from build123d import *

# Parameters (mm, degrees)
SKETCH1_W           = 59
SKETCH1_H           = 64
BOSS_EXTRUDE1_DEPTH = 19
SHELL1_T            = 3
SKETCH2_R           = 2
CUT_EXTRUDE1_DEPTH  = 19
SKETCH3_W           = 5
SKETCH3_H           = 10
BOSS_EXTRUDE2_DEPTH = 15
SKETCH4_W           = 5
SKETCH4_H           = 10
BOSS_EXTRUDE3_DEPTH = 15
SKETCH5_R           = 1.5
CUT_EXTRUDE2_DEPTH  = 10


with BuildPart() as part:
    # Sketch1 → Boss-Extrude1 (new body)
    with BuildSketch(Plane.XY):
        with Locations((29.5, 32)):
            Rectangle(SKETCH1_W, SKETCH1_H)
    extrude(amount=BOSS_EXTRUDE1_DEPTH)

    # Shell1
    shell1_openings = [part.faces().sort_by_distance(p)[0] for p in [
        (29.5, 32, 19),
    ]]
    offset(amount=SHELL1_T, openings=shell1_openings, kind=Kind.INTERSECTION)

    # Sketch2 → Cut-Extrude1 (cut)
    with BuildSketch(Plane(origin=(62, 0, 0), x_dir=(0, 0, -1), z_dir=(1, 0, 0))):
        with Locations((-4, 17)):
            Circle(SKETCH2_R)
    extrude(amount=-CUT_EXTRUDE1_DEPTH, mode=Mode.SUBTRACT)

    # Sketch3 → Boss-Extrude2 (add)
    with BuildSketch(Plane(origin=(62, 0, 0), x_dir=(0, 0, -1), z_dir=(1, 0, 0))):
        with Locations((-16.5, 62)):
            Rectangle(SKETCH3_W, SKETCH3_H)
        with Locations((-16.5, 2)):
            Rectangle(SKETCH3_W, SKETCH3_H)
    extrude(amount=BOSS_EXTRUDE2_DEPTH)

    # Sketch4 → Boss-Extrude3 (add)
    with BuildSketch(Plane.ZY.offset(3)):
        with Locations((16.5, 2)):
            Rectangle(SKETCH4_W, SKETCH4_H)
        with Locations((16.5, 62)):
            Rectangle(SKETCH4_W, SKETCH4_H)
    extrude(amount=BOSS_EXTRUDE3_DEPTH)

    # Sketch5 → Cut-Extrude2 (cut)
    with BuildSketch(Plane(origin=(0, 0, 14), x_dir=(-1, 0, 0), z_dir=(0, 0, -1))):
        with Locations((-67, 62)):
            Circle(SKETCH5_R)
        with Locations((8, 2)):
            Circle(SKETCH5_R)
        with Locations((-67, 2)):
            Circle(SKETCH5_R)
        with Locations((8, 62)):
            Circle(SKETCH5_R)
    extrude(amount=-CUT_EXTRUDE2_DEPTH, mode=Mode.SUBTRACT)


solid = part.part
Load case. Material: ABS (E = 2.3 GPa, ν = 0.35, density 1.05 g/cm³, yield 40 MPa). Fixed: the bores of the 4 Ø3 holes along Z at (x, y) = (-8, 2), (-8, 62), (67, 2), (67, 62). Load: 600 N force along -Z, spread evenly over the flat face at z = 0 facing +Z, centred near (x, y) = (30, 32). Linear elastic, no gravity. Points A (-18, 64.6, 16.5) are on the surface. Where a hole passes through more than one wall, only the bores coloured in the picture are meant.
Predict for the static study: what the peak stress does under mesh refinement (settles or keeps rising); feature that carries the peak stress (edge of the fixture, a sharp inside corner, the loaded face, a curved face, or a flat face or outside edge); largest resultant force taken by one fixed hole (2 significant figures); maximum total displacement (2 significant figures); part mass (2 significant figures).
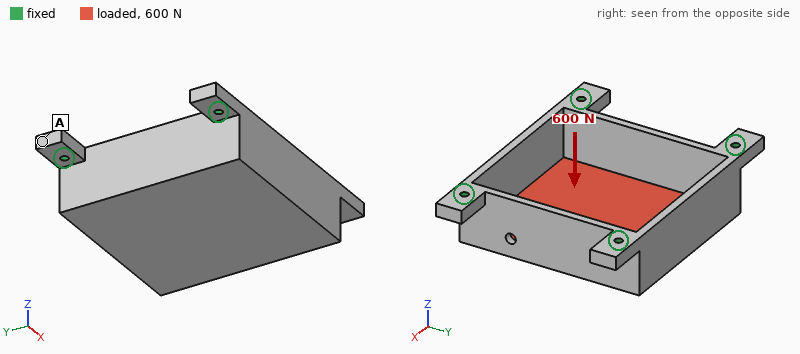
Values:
keeps rising
edge of the fixture
180 N
1.1 mm
33 g
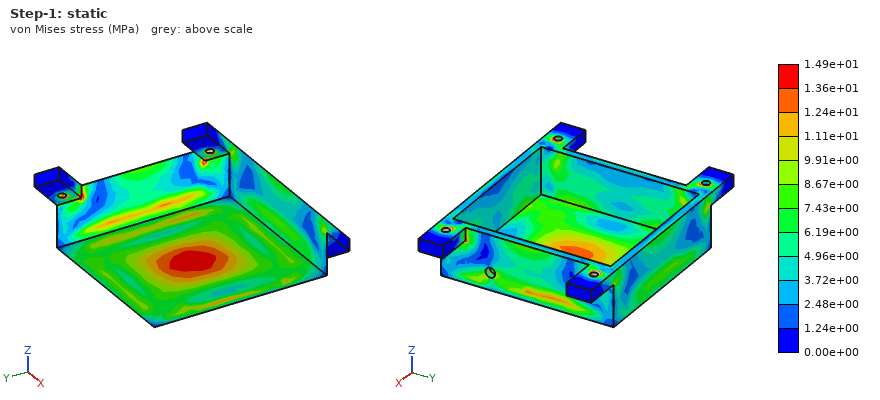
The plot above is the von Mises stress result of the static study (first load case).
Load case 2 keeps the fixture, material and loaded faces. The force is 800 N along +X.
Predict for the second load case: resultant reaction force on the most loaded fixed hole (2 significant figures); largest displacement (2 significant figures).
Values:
220 N
0.17 mm
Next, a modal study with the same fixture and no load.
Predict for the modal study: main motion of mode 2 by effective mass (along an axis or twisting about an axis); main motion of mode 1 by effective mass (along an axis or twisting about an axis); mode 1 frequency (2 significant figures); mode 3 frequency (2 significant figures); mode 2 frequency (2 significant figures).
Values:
along Y
along Z
1300 Hz
2100 Hz
1700 Hz
